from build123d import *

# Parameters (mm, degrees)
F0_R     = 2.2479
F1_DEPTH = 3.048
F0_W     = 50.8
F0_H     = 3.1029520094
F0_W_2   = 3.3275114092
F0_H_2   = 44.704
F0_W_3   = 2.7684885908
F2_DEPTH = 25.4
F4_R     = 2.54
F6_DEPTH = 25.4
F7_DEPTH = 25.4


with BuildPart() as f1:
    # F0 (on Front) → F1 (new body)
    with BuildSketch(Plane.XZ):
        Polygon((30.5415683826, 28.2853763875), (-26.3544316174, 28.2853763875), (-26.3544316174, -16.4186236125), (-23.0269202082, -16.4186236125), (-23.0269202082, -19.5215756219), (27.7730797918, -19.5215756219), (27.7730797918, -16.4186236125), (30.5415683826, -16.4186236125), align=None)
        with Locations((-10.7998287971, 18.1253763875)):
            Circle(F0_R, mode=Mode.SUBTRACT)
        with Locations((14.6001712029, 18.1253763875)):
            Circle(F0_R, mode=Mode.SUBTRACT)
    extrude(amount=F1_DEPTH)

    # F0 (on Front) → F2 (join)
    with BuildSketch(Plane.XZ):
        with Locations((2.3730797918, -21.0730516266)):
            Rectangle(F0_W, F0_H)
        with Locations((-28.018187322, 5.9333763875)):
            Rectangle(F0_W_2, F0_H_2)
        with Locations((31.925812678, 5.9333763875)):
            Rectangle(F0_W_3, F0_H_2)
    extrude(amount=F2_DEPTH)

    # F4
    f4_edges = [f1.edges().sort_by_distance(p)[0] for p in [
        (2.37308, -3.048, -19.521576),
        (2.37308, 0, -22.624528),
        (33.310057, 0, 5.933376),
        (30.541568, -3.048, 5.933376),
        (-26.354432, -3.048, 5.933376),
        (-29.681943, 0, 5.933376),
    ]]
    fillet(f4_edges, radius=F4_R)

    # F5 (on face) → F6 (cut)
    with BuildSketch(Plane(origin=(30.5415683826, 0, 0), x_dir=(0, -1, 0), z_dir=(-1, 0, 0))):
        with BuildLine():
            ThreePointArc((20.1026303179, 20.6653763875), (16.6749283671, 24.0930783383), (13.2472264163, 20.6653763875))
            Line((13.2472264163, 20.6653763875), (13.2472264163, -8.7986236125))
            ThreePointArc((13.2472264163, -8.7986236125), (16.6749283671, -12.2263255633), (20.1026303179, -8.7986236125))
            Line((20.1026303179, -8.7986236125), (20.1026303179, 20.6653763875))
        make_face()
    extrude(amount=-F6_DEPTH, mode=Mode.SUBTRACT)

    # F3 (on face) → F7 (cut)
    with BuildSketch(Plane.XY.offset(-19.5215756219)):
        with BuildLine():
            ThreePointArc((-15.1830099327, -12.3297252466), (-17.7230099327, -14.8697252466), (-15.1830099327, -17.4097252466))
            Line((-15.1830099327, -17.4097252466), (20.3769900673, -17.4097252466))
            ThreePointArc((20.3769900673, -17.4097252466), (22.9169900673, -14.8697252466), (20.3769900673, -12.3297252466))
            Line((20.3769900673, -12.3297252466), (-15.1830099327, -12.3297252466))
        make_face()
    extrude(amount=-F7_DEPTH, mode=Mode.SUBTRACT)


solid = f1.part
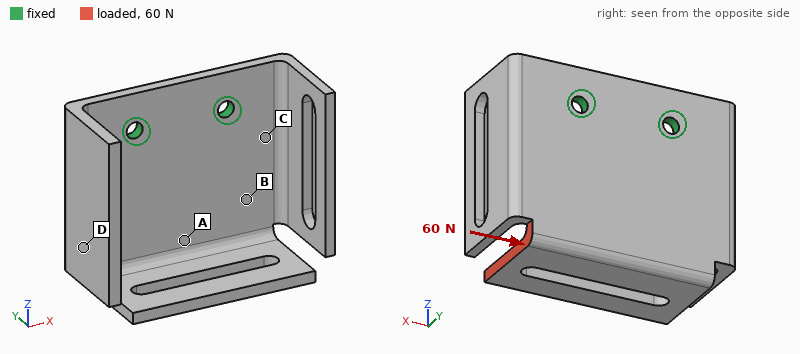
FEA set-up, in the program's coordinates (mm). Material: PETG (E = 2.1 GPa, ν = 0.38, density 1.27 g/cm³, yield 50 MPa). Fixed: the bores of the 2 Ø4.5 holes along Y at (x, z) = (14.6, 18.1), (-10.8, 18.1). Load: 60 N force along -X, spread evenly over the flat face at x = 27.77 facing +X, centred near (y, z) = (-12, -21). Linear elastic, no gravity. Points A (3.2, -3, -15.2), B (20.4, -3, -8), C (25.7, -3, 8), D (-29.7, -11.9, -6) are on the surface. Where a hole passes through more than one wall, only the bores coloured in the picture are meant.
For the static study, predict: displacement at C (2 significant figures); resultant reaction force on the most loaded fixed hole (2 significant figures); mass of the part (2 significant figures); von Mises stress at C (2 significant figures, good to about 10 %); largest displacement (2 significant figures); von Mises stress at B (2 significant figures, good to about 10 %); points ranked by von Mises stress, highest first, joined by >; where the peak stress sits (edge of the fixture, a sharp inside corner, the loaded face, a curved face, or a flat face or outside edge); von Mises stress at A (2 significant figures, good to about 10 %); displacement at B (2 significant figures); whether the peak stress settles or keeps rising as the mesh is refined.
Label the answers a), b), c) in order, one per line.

a) 0.18 mm
b) 88 N
c) 23 g
d) 1.4 MPa
e) 1.0 mm
f) 2.7 MPa
g) A > B > C > D
h) edge of the fixture
i) 3.5 MPa
j) 0.33 mm
k) keeps rising
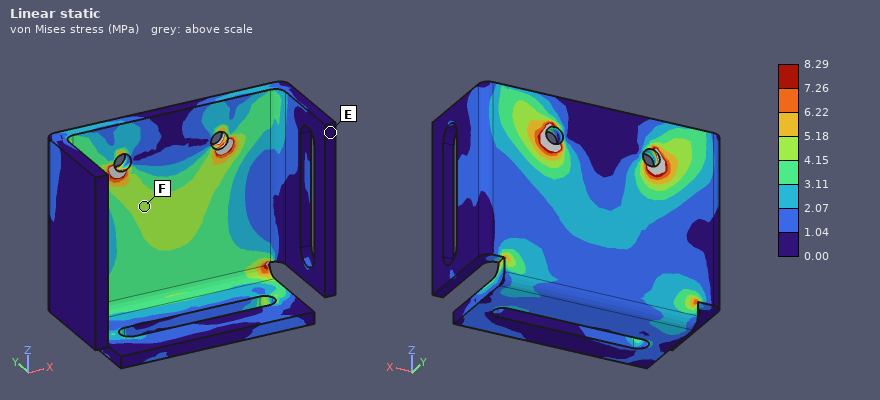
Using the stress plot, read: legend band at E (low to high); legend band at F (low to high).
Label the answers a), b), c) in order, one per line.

a) 0.00 to 1.04 MPa
b) 4.15 to 5.18 MPa
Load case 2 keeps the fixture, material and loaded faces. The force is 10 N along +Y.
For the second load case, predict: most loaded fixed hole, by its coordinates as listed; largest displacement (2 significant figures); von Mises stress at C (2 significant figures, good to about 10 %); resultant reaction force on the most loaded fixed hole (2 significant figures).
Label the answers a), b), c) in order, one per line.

a) (14.6, 18.1)
b) 0.86 mm
c) 1.1 MPa
d) 12 N
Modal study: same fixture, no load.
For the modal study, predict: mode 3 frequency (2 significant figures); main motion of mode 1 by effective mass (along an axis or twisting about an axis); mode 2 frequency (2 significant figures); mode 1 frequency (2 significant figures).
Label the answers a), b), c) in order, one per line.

a) 560 Hz
b) along Y
c) 340 Hz
d) 260 Hz
